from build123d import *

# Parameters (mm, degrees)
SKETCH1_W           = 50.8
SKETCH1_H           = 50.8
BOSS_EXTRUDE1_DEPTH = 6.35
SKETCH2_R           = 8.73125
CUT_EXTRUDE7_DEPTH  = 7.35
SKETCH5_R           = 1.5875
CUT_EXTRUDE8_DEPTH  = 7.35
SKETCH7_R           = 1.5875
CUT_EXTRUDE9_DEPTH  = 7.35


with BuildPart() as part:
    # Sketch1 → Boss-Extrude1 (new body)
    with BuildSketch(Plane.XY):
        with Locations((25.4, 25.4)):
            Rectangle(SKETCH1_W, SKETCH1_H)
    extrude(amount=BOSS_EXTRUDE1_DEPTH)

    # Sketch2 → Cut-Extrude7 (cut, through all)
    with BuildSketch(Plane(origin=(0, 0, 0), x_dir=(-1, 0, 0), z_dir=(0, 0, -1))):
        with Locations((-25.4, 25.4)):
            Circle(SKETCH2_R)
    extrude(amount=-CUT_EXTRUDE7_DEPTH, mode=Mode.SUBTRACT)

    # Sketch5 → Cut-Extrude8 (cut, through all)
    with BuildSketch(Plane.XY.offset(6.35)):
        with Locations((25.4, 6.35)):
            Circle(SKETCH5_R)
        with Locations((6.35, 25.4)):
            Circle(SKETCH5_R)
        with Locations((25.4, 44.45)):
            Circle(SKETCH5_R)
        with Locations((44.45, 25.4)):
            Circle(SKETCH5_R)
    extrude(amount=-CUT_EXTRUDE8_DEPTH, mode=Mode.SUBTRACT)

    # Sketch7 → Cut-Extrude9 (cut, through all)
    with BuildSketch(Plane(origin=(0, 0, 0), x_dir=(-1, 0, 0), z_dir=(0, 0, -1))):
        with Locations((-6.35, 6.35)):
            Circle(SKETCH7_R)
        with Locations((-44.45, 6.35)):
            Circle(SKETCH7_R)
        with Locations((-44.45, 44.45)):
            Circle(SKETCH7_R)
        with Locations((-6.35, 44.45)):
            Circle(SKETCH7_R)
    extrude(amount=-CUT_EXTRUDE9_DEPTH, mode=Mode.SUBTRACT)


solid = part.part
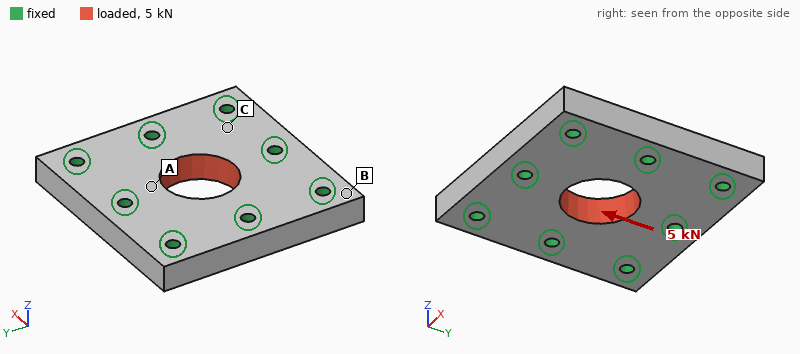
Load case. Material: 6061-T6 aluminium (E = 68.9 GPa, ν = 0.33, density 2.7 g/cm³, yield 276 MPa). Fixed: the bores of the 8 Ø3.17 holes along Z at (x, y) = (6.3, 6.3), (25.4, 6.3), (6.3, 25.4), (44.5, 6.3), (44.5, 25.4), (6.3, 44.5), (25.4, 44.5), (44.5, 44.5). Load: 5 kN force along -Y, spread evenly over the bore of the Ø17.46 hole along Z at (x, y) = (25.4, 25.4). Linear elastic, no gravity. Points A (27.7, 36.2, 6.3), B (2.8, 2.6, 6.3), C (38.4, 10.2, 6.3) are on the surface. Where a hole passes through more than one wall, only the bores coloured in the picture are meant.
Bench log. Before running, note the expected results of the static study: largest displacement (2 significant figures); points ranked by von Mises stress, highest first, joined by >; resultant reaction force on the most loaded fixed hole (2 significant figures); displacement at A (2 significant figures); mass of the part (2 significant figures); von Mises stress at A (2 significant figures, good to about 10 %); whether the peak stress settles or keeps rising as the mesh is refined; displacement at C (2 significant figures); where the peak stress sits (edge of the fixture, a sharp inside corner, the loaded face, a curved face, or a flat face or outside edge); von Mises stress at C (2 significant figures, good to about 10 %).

3.3 µm
A > C > B
1.2 kN
2.1 µm
39 g
16 MPa
keeps rising
1.0 µm
edge of the fixture
9.0 MPa
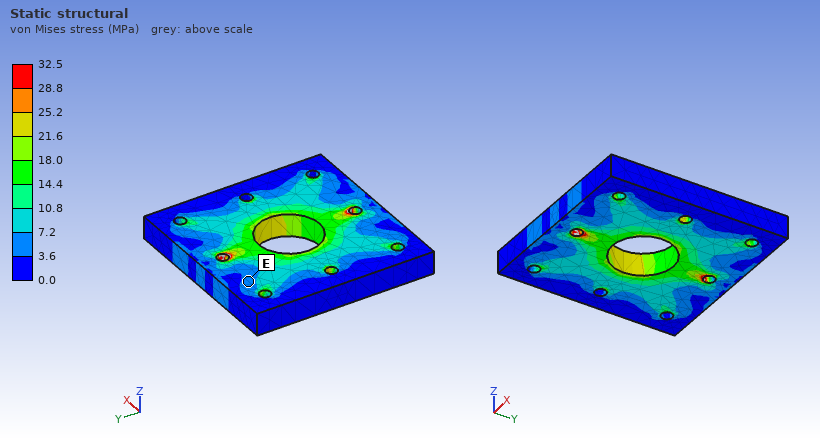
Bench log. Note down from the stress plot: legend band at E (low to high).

3.6 to 7.2 MPa
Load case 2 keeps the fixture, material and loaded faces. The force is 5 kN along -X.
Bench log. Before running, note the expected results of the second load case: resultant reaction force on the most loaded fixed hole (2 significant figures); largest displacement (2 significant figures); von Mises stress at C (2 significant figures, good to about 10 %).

1.2 kN
3.3 µm
9.1 MPa
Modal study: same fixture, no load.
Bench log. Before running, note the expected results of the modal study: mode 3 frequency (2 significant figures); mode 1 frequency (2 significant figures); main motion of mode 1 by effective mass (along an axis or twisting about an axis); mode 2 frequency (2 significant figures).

42 kHz
34 kHz
along Z
42 kHz
